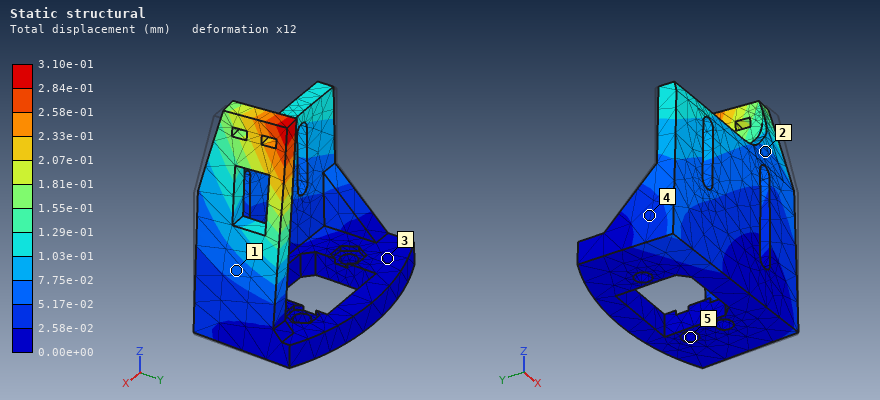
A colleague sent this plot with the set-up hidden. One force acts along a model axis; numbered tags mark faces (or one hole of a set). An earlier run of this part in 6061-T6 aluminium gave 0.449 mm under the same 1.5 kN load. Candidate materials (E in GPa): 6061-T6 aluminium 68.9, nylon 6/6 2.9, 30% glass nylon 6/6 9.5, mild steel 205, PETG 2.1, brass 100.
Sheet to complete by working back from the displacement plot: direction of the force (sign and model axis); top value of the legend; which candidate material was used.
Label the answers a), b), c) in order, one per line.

a) -X
b) 3.10e-01 mm
c) brass
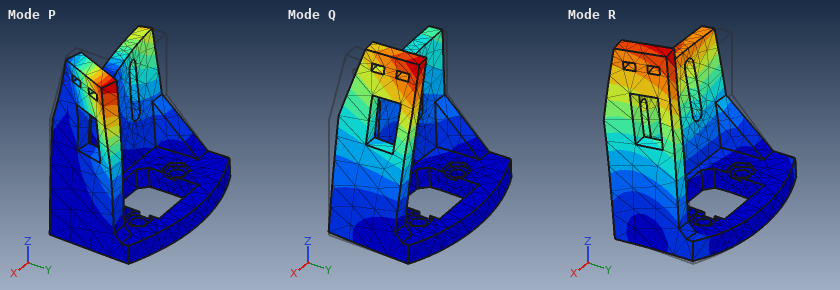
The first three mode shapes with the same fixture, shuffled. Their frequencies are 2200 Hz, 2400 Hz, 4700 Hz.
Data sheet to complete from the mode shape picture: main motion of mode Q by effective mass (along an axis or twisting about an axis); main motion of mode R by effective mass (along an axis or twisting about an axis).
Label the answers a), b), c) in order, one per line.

a) along X
b) along Y
